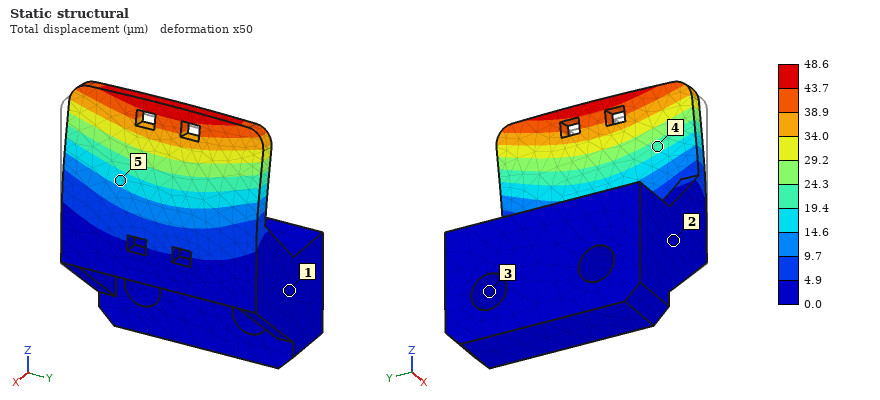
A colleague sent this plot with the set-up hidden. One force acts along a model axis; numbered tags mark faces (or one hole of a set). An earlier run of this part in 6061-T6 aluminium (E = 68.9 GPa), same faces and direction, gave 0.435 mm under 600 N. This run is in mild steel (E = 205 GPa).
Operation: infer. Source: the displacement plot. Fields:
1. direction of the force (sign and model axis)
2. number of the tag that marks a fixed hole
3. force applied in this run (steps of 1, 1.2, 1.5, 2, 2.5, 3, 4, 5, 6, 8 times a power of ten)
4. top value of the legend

-X
3
200 N
48.6 µm
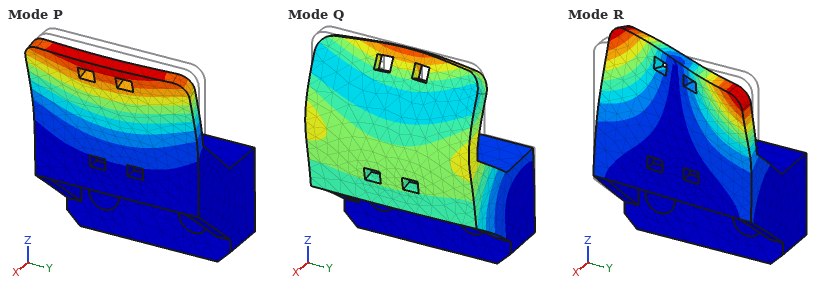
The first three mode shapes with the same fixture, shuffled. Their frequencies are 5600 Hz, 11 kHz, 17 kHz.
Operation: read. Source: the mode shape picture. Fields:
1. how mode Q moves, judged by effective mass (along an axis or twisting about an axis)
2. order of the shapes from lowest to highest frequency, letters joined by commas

along Z
P, R, Q
